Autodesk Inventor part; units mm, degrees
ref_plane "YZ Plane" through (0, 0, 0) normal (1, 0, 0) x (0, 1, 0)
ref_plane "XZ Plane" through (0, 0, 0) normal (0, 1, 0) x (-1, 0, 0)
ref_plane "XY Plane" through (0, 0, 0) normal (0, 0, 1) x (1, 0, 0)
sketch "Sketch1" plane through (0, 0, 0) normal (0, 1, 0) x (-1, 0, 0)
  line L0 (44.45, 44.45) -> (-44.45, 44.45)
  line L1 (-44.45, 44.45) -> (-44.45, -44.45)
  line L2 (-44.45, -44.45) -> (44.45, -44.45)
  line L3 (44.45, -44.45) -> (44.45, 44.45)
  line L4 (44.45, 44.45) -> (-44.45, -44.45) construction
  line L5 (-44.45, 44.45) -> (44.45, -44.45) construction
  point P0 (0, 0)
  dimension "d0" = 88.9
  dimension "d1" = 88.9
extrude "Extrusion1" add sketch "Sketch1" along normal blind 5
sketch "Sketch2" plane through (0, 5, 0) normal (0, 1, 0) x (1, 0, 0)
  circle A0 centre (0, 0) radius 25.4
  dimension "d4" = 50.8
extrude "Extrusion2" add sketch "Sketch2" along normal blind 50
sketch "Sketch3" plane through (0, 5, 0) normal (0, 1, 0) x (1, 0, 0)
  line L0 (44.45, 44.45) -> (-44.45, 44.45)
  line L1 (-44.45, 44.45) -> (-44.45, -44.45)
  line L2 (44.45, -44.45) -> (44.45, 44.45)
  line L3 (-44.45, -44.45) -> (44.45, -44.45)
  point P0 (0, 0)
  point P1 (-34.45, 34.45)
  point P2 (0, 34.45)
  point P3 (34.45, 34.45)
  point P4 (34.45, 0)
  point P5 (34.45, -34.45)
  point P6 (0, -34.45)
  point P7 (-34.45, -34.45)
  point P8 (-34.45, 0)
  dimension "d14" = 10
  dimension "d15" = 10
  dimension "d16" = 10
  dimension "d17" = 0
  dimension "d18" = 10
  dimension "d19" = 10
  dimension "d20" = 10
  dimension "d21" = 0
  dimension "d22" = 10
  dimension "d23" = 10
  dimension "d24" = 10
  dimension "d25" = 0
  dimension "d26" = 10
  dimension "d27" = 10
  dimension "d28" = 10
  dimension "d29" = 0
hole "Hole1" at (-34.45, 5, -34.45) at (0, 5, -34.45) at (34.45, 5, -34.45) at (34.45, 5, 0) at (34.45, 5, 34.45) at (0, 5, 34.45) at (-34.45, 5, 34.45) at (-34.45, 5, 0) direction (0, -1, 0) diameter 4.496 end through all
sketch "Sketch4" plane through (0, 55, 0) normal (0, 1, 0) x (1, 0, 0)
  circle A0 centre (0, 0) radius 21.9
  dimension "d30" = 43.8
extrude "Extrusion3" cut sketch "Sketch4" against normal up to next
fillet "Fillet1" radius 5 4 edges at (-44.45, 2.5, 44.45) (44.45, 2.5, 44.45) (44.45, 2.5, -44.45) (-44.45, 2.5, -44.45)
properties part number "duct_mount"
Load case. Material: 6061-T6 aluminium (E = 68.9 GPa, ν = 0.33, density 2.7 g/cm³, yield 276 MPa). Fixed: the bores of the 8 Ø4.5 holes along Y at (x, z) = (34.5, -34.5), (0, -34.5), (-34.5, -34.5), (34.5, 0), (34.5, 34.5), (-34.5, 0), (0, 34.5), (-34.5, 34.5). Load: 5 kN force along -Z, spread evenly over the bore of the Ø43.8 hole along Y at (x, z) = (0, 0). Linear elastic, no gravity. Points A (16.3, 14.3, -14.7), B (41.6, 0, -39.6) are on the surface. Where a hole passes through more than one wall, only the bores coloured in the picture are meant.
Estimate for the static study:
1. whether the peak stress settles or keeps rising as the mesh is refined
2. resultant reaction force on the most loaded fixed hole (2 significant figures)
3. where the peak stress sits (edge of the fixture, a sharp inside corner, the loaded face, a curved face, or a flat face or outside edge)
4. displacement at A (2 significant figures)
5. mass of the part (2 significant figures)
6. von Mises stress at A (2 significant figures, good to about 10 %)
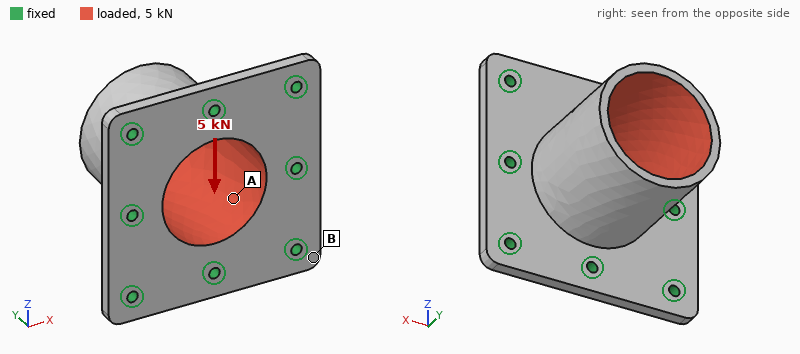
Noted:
keeps rising
2.1 kN
edge of the fixture
24 µm
150 g
24 MPa
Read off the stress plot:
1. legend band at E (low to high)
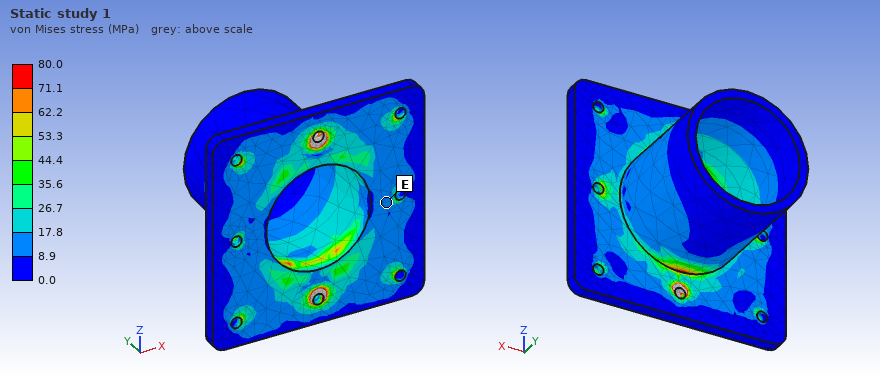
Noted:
8.9 to 17.8 MPa
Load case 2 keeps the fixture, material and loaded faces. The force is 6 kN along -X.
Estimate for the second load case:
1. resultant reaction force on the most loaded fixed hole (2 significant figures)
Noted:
2.5 kN
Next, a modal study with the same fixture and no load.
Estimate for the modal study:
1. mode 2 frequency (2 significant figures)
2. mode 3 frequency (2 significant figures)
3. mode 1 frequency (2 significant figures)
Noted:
4900 Hz
5000 Hz
4900 Hz
